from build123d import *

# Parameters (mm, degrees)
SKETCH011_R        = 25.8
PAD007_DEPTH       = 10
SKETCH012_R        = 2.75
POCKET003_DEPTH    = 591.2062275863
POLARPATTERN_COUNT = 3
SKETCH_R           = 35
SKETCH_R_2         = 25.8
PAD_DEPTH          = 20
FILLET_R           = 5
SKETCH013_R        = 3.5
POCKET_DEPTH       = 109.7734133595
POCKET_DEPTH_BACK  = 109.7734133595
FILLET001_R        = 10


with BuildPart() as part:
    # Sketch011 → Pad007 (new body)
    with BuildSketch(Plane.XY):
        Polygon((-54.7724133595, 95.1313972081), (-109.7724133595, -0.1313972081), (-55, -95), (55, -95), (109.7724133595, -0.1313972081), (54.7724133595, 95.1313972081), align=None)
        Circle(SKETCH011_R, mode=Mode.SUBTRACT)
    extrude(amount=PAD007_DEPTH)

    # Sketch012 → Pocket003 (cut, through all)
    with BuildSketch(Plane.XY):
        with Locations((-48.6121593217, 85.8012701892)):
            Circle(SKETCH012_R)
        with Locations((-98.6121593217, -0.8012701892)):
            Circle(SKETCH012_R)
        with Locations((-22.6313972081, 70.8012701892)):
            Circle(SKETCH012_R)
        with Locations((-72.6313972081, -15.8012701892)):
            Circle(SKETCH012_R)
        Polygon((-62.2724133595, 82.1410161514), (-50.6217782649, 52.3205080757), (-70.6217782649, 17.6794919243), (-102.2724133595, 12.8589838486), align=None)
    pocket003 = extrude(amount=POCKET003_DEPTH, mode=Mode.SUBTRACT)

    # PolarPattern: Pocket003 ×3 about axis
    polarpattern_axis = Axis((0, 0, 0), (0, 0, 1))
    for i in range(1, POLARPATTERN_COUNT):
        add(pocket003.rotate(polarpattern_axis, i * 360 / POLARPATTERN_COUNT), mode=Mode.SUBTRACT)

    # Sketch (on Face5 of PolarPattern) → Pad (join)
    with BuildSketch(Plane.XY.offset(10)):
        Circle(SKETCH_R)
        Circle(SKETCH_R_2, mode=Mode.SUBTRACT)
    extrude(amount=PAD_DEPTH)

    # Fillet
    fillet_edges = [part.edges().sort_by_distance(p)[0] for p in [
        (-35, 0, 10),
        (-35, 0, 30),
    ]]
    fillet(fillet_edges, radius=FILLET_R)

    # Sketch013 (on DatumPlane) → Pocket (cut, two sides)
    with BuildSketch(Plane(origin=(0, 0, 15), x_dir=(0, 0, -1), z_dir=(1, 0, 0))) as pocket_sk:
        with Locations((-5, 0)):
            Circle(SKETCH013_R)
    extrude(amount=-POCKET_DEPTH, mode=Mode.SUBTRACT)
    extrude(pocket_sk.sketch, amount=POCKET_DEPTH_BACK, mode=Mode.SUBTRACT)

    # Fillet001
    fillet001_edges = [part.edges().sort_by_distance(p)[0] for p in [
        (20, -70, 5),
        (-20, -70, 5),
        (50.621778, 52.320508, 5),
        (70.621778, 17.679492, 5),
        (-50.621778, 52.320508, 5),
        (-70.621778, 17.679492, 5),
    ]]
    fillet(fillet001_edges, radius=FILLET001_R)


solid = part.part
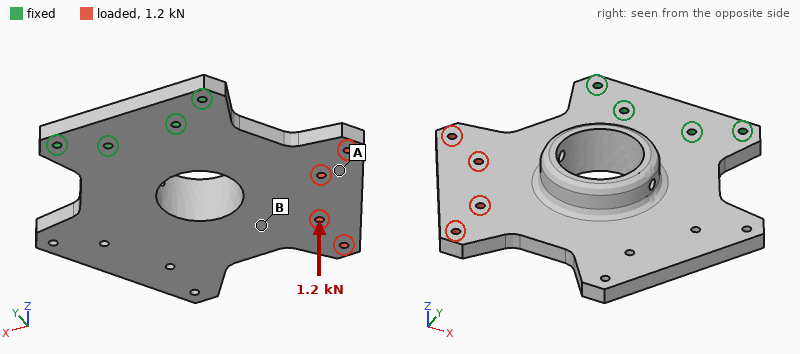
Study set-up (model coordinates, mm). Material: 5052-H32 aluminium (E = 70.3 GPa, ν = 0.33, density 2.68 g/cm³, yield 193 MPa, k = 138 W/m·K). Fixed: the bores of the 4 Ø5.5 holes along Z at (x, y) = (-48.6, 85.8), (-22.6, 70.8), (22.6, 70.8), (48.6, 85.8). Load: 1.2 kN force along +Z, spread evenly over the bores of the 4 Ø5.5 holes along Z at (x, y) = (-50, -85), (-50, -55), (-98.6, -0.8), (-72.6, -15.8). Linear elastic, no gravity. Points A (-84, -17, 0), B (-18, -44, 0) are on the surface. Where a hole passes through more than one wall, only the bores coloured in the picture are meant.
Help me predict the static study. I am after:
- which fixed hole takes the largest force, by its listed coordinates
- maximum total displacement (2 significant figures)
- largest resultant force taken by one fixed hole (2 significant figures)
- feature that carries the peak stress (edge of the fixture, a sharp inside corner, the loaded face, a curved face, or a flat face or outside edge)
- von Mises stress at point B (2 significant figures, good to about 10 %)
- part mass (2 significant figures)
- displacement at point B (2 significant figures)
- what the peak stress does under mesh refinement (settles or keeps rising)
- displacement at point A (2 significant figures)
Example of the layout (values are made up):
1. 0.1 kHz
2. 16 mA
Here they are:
1. (-22.6, 70.8)
2. 1.6 mm
3. 2.5 kN
4. edge of the fixture
5. 20 MPa
6. 750 g
7. 0.85 mm
8. keeps rising
9. 0.88 mm
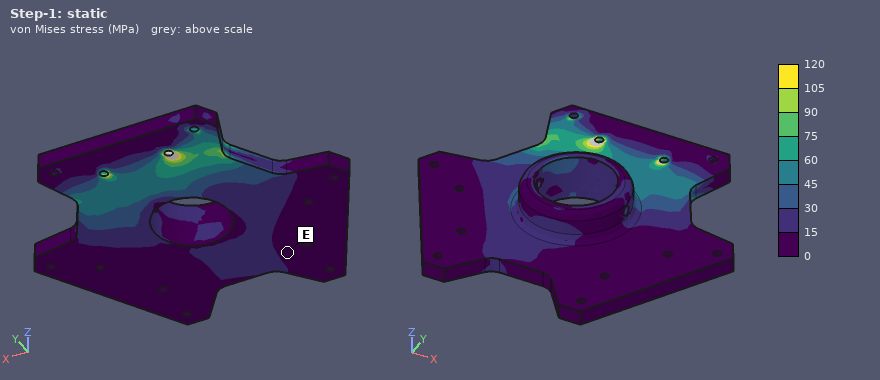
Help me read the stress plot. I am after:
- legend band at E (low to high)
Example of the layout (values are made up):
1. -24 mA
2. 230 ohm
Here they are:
1. 0 to 15 MPa
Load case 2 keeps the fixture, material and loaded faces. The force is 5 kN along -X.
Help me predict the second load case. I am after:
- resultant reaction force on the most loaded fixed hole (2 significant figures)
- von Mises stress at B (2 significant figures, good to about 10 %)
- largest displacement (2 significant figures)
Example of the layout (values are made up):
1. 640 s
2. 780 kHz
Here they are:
1. 4.3 kN
2. 10 MPa
3. 0.14 mm
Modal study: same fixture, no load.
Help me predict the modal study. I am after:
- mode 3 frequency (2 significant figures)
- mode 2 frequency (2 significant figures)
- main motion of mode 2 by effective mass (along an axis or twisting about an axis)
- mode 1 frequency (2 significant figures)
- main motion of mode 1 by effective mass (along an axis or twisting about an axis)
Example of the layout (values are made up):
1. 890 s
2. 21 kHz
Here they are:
1. 1600 Hz
2. 650 Hz
3. twisting about Y
4. 300 Hz
5. along Z
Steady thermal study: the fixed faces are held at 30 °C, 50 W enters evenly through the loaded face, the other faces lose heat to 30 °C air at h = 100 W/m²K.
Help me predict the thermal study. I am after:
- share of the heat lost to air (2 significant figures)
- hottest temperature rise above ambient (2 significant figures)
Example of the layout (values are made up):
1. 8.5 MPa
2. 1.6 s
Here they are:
1. 79 %
2. 22 K
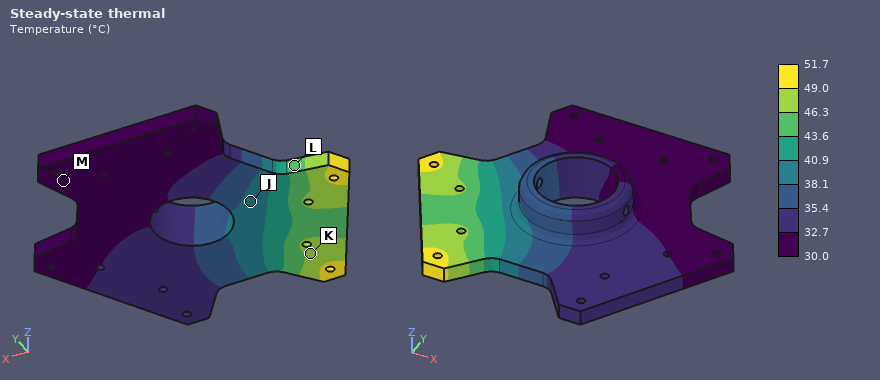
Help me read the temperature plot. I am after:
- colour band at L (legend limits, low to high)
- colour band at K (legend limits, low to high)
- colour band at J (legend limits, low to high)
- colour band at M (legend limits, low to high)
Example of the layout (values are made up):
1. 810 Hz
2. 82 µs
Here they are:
1. 43.6 to 46.3 °C
2. 46.3 to 49.0 °C
3. 38.1 to 40.9 °C
4. 30.0 to 32.7 °C
